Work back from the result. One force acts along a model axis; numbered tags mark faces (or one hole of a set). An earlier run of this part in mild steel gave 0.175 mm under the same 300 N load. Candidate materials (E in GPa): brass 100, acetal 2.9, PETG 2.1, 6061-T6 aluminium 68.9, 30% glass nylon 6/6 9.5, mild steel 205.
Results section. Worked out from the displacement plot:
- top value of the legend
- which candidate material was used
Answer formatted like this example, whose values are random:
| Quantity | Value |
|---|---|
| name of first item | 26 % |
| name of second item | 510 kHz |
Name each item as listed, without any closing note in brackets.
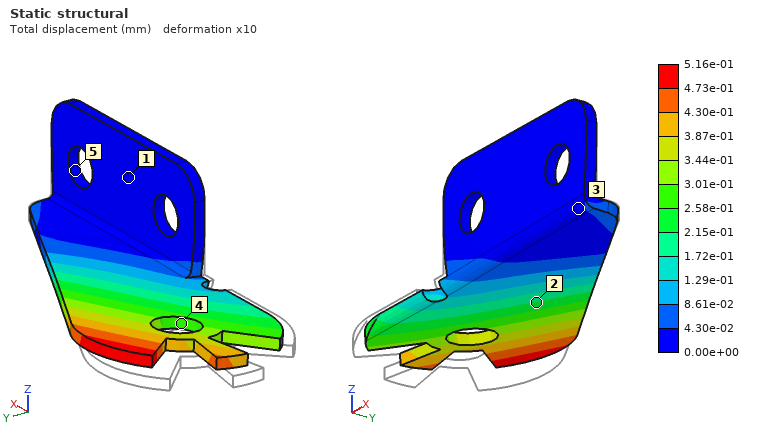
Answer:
| Quantity | Value |
|---|---|
| top value of the legend | 5.16e-01 mm |
| which candidate material was used | 6061-T6 aluminium |
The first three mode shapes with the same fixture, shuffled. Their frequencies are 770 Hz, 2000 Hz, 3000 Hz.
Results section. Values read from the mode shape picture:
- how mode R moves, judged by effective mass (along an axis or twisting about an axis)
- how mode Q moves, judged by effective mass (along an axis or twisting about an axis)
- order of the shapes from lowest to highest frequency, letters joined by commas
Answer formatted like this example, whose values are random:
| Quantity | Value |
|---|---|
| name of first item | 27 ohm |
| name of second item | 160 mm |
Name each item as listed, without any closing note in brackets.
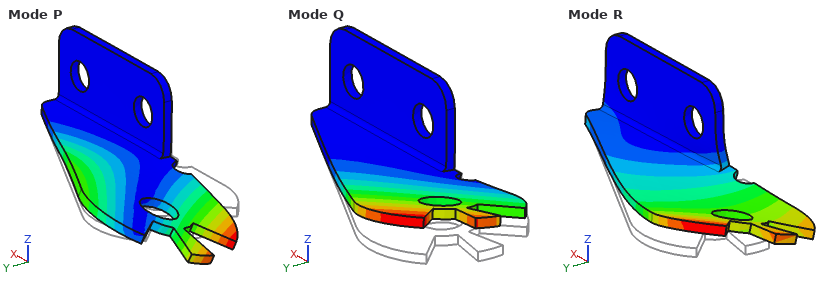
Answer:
| Quantity | Value |
|---|---|
| how mode R moves, judged by effective mass | along Y |
| how mode Q moves, judged by effective mass | along Z |
| order of the shapes from lowest to highest frequency, letters joined by commas | Q, P, R |
